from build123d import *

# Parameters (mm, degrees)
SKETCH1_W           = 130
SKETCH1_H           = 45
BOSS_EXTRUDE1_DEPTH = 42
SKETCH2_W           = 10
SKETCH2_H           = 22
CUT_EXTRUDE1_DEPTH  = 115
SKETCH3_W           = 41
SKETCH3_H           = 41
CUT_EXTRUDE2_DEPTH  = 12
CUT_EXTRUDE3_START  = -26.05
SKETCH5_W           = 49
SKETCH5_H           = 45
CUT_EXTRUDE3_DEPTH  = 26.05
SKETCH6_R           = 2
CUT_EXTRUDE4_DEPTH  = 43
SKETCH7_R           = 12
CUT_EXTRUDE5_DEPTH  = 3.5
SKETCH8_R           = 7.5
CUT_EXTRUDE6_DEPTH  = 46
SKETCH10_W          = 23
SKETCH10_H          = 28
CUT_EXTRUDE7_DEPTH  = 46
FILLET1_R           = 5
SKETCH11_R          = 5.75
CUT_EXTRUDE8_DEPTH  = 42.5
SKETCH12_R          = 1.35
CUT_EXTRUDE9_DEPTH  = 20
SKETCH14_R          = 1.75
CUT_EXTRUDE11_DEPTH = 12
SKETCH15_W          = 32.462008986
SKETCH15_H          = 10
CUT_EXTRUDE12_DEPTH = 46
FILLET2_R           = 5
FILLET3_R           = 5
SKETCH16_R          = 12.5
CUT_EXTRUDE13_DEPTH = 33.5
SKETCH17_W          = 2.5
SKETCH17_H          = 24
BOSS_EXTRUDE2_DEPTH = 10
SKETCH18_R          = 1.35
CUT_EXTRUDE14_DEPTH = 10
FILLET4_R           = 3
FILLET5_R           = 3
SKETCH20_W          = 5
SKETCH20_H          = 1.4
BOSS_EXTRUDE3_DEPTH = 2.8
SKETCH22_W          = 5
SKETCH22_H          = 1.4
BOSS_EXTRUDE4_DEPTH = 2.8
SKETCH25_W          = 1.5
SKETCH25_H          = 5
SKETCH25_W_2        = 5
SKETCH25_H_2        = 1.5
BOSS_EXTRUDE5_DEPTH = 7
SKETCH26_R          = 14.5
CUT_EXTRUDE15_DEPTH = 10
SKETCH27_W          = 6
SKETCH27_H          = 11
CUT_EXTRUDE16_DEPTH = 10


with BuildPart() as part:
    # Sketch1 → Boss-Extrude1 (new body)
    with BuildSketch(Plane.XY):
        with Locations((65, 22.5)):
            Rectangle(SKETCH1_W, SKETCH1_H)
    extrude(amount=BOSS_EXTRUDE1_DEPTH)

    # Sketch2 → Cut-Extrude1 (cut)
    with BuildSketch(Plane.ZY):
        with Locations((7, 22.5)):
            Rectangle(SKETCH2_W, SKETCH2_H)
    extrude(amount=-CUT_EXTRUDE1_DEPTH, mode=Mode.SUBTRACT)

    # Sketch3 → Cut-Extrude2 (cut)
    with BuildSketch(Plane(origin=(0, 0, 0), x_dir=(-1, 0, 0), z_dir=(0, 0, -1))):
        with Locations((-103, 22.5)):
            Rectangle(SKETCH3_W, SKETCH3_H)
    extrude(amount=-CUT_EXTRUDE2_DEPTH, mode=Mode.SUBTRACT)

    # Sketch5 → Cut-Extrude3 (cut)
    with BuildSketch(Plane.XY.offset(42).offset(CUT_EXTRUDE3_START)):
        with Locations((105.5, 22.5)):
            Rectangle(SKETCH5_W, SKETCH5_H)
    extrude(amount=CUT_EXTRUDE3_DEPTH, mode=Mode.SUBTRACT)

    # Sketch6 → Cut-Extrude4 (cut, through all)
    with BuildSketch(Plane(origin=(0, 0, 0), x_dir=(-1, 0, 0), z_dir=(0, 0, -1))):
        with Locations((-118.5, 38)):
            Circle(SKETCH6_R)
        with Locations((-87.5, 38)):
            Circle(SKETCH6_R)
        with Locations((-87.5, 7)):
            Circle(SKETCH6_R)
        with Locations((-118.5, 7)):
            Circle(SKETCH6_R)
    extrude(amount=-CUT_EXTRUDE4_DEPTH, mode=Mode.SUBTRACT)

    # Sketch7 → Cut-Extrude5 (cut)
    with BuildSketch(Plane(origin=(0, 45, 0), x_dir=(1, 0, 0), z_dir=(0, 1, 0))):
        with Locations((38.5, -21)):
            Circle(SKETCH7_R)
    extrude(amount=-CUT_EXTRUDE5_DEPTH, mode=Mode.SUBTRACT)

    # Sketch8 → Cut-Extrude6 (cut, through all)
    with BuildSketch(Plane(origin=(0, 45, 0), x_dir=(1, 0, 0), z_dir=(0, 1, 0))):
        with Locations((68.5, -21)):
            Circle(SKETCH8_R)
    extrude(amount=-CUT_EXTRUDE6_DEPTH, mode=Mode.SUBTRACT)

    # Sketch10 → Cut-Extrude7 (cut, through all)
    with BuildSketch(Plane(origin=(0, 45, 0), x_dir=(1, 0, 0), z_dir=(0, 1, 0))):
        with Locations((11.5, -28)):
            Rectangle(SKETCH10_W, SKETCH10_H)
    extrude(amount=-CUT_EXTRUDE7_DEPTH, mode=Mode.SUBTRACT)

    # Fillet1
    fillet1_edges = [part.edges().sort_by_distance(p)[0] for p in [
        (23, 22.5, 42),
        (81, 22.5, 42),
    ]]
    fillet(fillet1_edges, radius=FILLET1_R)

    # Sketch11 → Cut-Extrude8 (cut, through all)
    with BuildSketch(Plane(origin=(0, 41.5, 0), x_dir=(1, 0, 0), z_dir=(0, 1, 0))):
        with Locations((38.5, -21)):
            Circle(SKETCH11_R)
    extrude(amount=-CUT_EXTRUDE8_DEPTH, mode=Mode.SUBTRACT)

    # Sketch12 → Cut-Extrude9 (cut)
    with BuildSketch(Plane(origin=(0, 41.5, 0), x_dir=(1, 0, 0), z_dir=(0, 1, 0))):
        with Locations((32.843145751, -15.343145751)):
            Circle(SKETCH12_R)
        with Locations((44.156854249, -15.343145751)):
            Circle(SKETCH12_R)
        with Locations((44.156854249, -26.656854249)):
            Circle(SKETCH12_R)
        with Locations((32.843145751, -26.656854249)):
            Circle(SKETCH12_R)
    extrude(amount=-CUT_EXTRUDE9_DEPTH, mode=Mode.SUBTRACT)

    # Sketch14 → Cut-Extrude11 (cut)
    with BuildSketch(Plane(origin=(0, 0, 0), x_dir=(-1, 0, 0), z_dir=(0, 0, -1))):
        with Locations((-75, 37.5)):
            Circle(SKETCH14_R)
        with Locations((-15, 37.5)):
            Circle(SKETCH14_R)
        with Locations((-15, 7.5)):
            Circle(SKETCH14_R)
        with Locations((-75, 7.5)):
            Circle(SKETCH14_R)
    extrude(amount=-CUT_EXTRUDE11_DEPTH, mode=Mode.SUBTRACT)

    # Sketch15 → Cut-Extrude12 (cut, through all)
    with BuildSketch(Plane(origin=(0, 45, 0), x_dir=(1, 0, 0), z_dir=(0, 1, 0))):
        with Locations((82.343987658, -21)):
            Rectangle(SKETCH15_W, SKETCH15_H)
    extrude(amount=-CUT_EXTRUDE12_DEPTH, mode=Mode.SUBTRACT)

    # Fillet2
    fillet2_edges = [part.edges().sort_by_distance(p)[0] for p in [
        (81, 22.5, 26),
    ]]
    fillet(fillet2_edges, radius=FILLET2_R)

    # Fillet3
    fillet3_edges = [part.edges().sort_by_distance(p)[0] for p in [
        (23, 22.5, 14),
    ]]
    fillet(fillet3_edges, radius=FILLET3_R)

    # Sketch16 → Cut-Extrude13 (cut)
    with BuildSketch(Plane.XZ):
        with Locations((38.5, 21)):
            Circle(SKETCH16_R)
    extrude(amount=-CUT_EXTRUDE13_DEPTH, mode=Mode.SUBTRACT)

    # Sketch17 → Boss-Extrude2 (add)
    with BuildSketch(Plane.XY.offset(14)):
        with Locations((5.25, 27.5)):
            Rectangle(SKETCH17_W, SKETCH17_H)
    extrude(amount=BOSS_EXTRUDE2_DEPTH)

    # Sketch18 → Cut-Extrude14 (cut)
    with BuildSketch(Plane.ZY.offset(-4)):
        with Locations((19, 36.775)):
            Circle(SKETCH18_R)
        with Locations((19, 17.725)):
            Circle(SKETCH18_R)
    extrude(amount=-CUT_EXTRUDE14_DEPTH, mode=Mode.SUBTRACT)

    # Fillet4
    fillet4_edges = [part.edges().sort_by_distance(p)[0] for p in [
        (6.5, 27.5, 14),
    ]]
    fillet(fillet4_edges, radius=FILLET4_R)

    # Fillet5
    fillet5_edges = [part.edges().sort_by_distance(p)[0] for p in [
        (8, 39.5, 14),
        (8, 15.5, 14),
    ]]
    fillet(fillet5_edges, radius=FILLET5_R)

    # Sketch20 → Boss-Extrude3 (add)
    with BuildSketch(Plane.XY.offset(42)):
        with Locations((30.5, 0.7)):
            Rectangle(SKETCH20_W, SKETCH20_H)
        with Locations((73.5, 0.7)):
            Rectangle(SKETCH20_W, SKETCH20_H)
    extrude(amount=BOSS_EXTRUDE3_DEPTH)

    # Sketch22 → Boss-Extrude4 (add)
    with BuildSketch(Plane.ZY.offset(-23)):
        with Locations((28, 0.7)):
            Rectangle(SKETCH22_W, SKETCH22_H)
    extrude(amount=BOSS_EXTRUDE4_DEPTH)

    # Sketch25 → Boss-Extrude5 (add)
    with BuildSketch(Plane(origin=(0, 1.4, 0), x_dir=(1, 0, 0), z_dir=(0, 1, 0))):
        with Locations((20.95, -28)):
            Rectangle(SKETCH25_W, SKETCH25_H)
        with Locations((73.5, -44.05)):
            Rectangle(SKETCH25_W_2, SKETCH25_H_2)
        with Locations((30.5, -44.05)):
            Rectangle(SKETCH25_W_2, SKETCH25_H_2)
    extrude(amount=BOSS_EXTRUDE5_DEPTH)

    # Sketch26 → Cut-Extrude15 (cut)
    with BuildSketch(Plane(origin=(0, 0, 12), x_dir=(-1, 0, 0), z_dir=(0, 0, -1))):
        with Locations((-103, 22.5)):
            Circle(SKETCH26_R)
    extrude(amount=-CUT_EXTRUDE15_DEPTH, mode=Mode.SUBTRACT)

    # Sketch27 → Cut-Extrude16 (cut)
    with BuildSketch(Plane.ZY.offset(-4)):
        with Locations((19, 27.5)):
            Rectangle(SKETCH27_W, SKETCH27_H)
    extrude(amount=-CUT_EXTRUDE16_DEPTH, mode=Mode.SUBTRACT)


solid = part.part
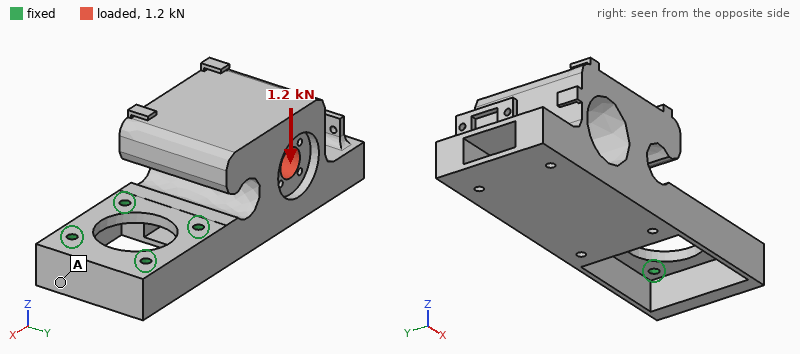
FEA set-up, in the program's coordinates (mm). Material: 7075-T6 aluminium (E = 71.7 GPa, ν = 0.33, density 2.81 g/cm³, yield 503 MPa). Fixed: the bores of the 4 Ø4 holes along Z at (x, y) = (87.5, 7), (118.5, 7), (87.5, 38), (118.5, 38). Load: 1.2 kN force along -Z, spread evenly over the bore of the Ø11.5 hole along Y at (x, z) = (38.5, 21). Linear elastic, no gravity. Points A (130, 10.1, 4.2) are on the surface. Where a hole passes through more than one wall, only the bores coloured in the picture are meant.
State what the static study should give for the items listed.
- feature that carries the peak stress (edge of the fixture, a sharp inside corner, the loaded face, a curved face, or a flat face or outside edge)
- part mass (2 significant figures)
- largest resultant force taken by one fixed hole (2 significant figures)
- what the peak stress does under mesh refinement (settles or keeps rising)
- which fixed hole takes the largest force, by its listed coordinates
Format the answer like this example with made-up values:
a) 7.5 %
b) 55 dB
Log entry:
a) edge of the fixture
b) 250 g
c) 2.1 kN
d) keeps rising
e) (87.5, 38)
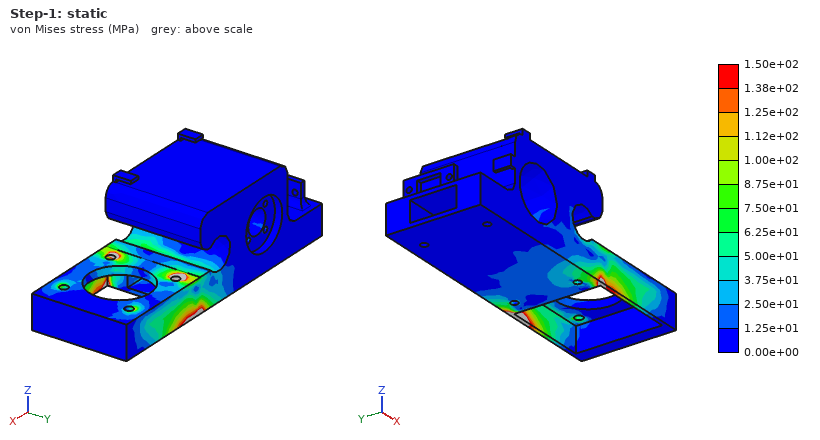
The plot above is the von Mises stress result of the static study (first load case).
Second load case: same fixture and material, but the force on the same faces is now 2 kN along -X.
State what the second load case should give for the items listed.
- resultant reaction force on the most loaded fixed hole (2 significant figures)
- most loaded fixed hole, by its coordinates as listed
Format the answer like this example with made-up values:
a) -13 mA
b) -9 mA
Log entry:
a) 1.9 kN
b) (87.5, 38)
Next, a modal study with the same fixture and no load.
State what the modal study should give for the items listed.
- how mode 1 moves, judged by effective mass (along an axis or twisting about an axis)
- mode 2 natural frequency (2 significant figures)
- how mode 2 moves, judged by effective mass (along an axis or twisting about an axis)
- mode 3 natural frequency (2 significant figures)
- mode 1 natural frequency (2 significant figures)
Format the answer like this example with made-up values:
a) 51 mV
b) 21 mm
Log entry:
a) along Z
b) 1800 Hz
c) along Y
d) 3000 Hz
e) 670 Hz
